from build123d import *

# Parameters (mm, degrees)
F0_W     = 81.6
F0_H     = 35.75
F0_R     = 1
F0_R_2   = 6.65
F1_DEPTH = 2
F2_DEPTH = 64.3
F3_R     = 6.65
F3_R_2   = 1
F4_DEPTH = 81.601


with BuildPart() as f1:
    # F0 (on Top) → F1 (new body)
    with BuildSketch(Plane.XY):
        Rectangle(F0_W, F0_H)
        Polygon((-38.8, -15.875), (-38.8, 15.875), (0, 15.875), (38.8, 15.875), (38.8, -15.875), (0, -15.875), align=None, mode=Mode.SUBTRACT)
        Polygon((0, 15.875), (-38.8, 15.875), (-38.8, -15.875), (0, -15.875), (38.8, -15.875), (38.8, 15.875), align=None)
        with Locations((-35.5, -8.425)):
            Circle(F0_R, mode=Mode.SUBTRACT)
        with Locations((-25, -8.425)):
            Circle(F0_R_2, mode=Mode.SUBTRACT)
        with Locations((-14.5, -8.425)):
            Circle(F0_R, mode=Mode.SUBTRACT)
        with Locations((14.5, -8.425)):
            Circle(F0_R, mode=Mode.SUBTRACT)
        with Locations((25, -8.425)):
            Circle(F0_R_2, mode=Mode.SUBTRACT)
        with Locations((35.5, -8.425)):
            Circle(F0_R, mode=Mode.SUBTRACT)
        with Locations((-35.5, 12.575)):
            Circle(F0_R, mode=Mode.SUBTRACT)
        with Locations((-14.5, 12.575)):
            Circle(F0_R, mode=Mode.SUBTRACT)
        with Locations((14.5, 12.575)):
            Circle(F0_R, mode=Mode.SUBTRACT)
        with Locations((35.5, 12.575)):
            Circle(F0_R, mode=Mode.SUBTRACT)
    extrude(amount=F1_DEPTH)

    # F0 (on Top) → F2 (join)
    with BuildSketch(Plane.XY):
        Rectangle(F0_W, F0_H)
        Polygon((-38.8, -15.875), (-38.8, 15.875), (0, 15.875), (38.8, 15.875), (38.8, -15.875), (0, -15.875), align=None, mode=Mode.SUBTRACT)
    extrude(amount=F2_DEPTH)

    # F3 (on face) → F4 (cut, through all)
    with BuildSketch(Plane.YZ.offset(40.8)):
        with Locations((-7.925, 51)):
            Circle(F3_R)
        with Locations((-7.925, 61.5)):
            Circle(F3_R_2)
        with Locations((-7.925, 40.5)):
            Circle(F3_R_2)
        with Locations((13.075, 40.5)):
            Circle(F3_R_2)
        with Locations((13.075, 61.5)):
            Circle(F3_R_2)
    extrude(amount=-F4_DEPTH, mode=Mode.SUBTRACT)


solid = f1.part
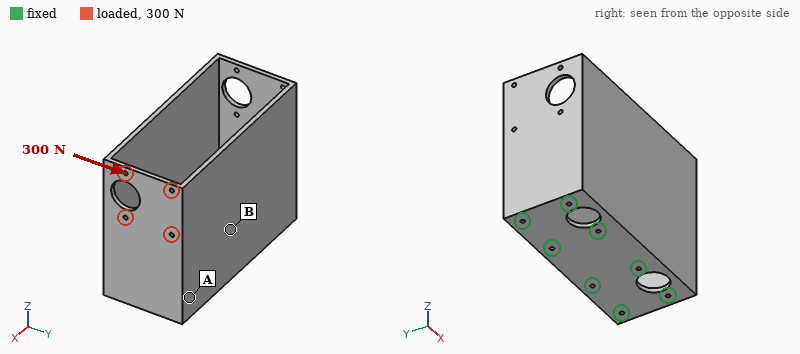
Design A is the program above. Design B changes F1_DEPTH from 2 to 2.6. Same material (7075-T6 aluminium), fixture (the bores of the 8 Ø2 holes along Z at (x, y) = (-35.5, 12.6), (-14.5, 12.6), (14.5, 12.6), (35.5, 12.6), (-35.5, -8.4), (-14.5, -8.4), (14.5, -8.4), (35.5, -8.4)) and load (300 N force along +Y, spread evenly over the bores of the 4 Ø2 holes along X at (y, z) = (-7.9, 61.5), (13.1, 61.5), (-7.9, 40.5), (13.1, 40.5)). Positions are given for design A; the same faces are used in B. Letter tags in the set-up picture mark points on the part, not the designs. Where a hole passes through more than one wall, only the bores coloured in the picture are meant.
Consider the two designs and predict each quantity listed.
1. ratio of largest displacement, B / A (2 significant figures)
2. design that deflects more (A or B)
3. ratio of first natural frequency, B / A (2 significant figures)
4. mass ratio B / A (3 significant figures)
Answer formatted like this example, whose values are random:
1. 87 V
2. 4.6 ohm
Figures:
1. 0.72
2. A
3. 1.0
4. 1.04
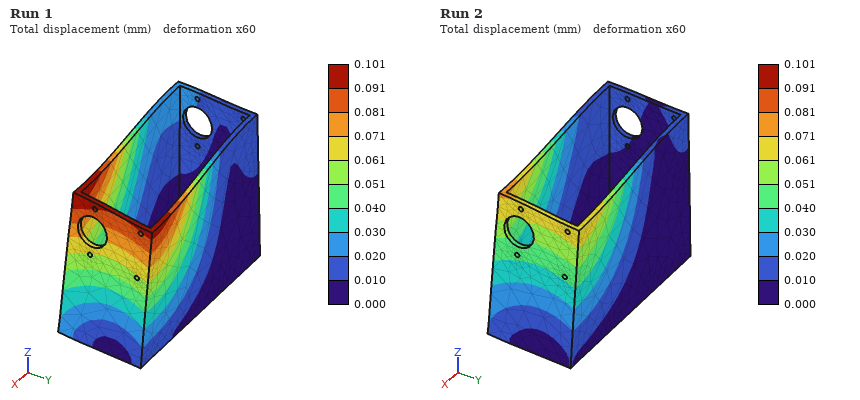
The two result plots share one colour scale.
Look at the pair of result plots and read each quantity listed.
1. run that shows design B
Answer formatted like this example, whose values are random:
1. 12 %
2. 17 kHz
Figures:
1. Run 2
